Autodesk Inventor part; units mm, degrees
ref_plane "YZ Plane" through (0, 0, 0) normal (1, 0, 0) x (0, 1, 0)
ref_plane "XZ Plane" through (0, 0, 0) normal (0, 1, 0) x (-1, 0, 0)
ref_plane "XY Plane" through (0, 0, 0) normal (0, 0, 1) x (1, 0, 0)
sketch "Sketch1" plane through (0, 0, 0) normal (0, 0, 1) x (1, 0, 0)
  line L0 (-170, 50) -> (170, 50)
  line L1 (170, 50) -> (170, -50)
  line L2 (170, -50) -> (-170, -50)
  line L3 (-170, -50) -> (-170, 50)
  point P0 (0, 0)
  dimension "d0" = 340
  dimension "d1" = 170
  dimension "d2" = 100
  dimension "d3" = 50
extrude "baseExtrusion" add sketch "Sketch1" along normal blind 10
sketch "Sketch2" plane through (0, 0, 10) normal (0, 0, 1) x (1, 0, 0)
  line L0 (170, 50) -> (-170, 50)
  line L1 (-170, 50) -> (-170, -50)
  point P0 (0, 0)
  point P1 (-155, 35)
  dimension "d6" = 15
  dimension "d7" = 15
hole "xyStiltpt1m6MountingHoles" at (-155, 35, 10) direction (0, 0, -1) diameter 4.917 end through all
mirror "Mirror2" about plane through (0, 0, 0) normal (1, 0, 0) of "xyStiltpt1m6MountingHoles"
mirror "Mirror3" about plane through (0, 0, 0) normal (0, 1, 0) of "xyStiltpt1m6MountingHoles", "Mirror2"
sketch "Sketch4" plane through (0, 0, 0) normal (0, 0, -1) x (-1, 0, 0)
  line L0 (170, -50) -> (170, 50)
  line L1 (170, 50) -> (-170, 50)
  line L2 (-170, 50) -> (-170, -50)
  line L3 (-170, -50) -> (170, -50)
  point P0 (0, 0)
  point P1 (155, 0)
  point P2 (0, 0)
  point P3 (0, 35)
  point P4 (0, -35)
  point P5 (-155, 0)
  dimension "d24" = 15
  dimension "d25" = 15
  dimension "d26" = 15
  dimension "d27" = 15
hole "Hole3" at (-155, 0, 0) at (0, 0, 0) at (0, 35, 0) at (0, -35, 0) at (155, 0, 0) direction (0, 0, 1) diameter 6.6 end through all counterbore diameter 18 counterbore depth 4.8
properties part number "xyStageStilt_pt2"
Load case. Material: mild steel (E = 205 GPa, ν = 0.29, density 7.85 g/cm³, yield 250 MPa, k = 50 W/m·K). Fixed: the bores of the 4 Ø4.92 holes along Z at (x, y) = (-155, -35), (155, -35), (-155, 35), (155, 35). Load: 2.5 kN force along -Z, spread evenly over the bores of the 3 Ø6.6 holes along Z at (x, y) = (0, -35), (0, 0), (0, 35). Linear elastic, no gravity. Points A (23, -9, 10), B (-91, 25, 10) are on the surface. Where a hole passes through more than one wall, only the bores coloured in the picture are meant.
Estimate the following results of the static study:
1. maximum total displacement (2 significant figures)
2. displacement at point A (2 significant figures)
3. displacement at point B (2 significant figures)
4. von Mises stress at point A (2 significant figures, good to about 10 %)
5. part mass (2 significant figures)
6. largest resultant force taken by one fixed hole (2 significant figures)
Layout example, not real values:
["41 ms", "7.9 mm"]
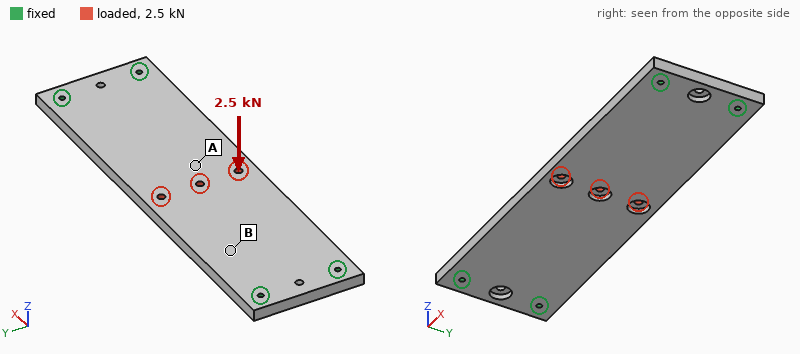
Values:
["0.30 mm", "0.27 mm", "0.11 mm", "41 MPa", "2.6 kg", "720 N"]
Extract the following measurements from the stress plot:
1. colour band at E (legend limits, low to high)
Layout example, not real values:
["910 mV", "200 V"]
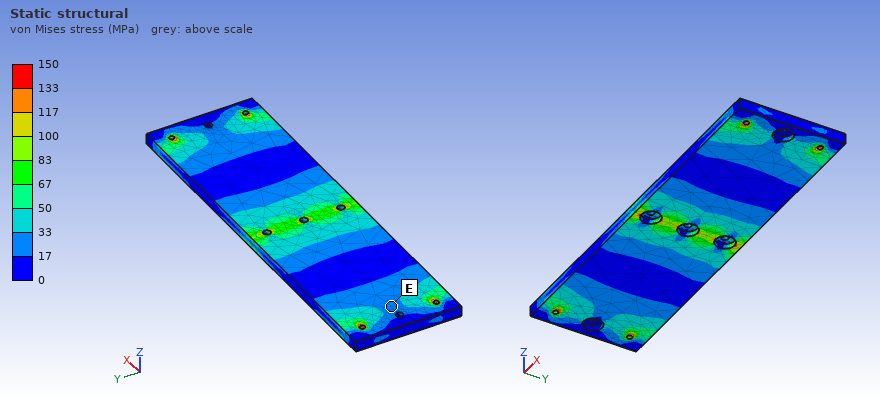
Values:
["17 to 33 MPa"]
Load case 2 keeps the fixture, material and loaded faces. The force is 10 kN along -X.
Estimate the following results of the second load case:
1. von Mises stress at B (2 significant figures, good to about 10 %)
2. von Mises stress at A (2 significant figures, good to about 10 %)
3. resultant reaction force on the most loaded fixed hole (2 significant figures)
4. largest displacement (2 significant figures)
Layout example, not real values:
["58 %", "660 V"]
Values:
["6.2 MPa", "10.0 MPa", "2.5 kN", "7.8 µm"]
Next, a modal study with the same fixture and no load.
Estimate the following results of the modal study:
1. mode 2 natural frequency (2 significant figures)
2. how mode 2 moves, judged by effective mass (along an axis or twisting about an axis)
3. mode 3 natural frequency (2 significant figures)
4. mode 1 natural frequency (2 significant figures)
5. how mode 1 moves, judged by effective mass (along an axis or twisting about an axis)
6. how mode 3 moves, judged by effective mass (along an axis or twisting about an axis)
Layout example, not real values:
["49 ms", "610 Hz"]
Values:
["1200 Hz", "twisting about X", "1400 Hz", "490 Hz", "along Z", "twisting about Y"]
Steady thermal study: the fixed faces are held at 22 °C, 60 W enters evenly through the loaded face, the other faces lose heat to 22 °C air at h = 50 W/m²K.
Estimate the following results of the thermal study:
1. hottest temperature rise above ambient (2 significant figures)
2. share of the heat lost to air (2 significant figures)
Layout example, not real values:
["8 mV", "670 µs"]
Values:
["50 K", "84 %"]
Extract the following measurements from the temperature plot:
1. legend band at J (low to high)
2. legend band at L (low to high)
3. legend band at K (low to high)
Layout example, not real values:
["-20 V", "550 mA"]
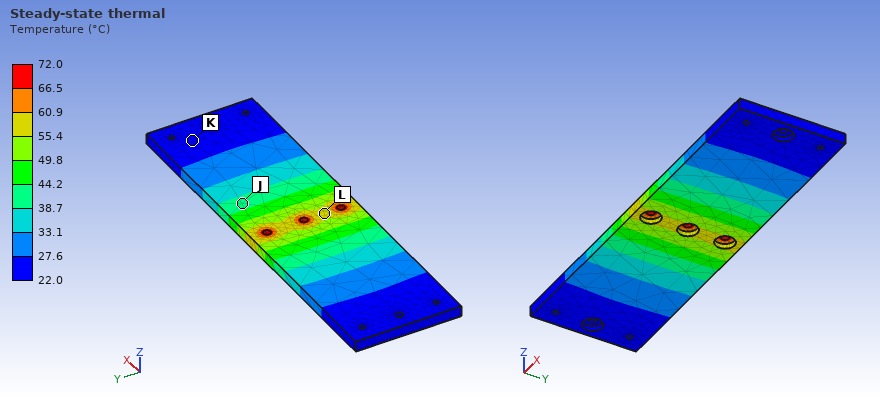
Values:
["38.7 to 44.2 °C", "55.4 to 60.9 °C", "22.0 to 27.6 °C"]
